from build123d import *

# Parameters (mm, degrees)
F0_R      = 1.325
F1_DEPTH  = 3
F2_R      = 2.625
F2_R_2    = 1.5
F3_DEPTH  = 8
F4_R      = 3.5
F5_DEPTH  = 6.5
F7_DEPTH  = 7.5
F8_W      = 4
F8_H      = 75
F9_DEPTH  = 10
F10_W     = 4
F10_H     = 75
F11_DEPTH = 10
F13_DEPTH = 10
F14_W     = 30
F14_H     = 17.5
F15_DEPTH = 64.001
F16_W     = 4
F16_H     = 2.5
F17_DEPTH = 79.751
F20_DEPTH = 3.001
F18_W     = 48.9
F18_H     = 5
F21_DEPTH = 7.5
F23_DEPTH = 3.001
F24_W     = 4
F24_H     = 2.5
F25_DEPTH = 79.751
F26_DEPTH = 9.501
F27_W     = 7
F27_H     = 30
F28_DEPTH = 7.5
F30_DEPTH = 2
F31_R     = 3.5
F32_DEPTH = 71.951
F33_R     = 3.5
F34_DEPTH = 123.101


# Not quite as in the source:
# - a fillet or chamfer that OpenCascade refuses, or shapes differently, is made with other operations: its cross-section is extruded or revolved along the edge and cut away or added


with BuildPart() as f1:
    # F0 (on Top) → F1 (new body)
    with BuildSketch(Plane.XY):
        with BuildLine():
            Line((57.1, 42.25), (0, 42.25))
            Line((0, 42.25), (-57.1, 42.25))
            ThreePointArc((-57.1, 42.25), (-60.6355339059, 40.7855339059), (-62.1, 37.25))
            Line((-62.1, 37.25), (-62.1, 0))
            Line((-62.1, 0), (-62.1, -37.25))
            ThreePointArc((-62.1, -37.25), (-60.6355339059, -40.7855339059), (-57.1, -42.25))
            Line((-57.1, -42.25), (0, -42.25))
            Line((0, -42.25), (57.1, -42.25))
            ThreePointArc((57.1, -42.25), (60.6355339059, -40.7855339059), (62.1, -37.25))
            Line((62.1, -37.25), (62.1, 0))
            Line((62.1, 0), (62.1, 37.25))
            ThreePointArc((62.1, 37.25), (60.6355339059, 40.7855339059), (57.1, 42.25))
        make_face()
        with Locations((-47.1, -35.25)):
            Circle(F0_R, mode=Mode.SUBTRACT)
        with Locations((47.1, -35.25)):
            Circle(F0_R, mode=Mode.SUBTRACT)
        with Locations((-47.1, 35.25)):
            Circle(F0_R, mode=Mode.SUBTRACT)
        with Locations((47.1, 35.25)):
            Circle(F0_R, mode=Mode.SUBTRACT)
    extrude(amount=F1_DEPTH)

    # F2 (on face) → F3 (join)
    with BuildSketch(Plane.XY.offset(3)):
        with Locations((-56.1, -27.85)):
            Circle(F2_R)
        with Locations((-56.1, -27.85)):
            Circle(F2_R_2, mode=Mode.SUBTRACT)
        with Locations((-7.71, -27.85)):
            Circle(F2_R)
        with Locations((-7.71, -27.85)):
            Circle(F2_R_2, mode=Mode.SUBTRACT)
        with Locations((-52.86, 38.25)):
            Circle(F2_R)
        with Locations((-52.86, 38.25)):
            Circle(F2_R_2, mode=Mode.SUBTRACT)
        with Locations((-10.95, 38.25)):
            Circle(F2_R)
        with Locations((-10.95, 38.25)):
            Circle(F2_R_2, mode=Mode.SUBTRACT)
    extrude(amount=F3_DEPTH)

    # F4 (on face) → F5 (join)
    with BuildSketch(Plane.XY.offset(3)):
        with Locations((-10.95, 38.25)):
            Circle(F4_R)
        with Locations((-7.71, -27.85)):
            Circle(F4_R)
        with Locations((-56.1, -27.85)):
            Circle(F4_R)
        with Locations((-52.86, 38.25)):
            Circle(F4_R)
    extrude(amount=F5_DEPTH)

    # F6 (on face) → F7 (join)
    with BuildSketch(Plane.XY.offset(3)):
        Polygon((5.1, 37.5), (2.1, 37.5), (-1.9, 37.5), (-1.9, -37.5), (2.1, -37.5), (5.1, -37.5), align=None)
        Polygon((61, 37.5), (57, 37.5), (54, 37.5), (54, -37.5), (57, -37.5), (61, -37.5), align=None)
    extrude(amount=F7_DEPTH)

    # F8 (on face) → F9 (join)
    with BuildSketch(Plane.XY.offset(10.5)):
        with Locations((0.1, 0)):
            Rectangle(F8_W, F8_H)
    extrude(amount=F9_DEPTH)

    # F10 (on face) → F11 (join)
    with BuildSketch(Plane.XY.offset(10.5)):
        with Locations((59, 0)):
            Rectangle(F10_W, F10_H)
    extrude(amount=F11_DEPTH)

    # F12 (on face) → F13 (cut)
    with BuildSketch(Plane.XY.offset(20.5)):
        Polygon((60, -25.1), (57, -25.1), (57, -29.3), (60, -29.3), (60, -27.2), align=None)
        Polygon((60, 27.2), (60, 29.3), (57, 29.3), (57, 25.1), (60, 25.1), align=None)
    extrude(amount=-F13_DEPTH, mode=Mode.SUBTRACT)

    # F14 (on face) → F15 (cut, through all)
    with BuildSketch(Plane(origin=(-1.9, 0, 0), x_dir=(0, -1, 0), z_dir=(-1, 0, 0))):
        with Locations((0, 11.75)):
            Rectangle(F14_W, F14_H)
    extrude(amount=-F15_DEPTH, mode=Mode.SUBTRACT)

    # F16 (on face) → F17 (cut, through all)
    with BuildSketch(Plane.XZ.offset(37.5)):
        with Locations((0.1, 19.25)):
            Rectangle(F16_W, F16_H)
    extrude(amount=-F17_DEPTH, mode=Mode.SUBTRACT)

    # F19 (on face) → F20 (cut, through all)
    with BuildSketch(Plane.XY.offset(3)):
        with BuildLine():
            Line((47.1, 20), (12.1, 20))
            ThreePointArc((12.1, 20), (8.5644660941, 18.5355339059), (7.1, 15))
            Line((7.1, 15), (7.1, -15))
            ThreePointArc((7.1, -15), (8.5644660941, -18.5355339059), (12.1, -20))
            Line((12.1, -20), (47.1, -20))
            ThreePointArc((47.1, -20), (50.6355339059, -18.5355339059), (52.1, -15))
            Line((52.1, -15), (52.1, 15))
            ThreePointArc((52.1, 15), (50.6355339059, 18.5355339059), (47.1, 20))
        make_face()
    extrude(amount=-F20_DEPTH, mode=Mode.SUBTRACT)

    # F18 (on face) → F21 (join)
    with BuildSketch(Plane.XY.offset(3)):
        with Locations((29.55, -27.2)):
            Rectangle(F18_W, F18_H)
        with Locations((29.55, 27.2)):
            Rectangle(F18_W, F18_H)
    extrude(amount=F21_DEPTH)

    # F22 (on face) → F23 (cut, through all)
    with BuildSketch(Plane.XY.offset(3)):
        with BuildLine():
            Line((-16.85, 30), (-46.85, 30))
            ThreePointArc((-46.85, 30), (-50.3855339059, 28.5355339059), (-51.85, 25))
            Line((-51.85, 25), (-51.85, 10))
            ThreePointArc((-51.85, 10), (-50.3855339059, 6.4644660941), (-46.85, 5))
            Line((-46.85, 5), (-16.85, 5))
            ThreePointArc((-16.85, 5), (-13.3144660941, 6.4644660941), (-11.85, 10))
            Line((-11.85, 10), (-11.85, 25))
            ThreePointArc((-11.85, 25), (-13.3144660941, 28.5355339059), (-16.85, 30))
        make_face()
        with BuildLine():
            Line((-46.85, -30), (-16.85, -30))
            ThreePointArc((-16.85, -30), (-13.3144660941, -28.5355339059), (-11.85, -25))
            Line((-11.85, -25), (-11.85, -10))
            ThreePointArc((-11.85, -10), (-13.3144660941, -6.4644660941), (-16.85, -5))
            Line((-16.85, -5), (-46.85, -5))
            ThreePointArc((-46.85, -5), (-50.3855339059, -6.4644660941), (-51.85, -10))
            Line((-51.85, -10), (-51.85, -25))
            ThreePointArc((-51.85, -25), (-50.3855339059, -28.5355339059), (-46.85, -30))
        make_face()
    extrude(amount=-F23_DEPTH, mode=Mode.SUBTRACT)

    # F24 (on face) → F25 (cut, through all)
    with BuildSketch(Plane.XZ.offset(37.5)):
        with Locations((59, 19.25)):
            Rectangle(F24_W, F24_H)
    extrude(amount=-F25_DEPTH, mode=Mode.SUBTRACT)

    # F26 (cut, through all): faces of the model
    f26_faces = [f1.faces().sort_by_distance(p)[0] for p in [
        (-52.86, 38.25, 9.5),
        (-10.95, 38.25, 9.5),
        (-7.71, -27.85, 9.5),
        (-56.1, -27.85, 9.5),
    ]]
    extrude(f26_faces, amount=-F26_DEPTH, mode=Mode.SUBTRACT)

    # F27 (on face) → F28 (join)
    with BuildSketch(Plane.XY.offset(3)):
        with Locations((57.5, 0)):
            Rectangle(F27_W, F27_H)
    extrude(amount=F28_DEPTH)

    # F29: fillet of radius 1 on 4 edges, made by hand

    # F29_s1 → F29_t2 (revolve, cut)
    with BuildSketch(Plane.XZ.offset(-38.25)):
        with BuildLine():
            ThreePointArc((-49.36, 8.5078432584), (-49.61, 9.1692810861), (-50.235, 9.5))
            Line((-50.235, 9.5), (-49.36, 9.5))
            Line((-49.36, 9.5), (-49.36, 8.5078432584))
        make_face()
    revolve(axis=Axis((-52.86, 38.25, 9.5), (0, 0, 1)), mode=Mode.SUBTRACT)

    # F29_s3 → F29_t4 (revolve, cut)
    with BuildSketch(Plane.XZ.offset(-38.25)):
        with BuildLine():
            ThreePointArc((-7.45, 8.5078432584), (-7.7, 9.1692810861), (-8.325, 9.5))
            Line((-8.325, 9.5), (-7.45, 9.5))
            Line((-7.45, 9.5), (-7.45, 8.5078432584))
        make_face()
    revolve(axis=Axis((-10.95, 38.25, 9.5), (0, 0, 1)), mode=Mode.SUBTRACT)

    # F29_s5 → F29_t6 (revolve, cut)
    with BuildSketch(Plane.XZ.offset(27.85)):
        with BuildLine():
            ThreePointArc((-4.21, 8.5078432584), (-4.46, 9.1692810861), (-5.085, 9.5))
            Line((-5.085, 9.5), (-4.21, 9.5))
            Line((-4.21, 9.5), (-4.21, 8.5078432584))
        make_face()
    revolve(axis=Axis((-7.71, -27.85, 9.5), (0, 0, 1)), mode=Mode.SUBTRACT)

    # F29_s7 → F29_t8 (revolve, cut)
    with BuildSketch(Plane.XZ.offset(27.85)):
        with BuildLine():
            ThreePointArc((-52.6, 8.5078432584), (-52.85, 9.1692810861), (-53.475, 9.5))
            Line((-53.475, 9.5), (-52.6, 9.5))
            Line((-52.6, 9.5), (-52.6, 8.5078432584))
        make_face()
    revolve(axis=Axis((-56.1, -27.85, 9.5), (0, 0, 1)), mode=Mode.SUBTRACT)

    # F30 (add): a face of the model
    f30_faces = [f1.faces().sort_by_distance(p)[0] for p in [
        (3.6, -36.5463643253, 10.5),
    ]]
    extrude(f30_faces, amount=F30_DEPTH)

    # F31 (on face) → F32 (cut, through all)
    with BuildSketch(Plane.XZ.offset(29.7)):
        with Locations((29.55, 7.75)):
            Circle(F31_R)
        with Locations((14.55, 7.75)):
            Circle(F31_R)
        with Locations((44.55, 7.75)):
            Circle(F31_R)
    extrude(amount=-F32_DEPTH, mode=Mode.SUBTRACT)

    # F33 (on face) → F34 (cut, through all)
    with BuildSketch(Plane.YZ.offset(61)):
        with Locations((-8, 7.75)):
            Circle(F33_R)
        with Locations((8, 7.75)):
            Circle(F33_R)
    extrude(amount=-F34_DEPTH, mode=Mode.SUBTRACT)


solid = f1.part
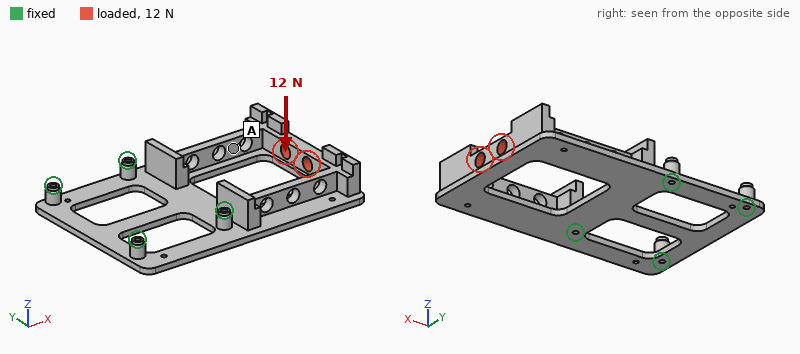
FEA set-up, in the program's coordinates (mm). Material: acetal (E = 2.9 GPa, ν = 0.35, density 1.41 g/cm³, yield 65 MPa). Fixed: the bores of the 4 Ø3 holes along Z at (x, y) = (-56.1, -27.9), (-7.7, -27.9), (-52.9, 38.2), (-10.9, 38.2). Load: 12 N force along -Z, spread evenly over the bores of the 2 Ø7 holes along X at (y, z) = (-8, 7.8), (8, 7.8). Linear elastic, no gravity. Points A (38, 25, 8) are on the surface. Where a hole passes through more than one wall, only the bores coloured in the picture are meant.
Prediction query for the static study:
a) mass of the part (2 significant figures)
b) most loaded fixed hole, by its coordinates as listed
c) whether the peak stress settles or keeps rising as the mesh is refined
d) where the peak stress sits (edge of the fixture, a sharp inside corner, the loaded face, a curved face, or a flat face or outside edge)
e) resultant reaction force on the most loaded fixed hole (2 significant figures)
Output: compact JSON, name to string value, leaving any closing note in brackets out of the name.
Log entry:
{"mass of the part": "48 g", "most loaded fixed hole, by its coordinates as listed": "(-7.7, -27.9)", "whether the peak stress settles or keeps rising as the mesh is refined": "keeps rising", "where the peak stress sits": "edge of the fixture", "resultant reaction force on the most loaded fixed hole": "11 N"}
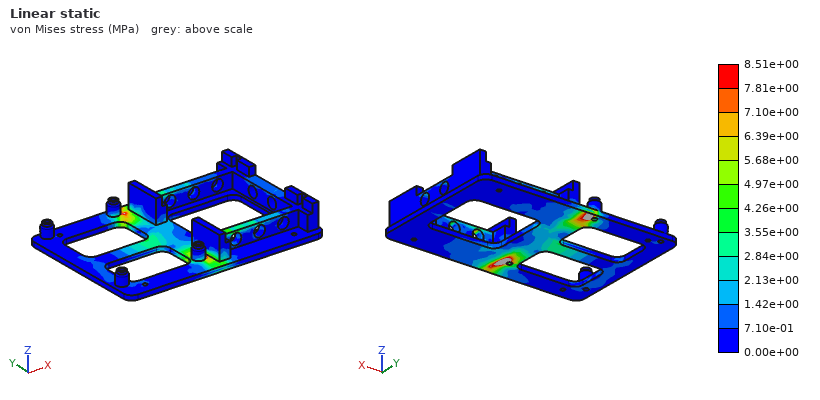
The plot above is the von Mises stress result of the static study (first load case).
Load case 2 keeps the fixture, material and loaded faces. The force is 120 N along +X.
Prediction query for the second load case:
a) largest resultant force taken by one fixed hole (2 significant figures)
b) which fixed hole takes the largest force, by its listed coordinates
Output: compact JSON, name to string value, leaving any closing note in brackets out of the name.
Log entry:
{"largest resultant force taken by one fixed hole": "60 N", "which fixed hole takes the largest force, by its listed coordinates": "(-7.7, -27.9)"}
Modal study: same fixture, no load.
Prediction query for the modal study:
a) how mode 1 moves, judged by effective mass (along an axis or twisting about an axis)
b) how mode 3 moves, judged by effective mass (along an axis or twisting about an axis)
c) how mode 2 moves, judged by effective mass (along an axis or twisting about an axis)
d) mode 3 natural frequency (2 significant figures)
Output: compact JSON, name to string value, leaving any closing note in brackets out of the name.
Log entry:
{"how mode 1 moves, judged by effective mass": "along Z", "how mode 3 moves, judged by effective mass": "along Y", "how mode 2 moves, judged by effective mass": "twisting about X", "mode 3 natural frequency": "750 Hz"}
